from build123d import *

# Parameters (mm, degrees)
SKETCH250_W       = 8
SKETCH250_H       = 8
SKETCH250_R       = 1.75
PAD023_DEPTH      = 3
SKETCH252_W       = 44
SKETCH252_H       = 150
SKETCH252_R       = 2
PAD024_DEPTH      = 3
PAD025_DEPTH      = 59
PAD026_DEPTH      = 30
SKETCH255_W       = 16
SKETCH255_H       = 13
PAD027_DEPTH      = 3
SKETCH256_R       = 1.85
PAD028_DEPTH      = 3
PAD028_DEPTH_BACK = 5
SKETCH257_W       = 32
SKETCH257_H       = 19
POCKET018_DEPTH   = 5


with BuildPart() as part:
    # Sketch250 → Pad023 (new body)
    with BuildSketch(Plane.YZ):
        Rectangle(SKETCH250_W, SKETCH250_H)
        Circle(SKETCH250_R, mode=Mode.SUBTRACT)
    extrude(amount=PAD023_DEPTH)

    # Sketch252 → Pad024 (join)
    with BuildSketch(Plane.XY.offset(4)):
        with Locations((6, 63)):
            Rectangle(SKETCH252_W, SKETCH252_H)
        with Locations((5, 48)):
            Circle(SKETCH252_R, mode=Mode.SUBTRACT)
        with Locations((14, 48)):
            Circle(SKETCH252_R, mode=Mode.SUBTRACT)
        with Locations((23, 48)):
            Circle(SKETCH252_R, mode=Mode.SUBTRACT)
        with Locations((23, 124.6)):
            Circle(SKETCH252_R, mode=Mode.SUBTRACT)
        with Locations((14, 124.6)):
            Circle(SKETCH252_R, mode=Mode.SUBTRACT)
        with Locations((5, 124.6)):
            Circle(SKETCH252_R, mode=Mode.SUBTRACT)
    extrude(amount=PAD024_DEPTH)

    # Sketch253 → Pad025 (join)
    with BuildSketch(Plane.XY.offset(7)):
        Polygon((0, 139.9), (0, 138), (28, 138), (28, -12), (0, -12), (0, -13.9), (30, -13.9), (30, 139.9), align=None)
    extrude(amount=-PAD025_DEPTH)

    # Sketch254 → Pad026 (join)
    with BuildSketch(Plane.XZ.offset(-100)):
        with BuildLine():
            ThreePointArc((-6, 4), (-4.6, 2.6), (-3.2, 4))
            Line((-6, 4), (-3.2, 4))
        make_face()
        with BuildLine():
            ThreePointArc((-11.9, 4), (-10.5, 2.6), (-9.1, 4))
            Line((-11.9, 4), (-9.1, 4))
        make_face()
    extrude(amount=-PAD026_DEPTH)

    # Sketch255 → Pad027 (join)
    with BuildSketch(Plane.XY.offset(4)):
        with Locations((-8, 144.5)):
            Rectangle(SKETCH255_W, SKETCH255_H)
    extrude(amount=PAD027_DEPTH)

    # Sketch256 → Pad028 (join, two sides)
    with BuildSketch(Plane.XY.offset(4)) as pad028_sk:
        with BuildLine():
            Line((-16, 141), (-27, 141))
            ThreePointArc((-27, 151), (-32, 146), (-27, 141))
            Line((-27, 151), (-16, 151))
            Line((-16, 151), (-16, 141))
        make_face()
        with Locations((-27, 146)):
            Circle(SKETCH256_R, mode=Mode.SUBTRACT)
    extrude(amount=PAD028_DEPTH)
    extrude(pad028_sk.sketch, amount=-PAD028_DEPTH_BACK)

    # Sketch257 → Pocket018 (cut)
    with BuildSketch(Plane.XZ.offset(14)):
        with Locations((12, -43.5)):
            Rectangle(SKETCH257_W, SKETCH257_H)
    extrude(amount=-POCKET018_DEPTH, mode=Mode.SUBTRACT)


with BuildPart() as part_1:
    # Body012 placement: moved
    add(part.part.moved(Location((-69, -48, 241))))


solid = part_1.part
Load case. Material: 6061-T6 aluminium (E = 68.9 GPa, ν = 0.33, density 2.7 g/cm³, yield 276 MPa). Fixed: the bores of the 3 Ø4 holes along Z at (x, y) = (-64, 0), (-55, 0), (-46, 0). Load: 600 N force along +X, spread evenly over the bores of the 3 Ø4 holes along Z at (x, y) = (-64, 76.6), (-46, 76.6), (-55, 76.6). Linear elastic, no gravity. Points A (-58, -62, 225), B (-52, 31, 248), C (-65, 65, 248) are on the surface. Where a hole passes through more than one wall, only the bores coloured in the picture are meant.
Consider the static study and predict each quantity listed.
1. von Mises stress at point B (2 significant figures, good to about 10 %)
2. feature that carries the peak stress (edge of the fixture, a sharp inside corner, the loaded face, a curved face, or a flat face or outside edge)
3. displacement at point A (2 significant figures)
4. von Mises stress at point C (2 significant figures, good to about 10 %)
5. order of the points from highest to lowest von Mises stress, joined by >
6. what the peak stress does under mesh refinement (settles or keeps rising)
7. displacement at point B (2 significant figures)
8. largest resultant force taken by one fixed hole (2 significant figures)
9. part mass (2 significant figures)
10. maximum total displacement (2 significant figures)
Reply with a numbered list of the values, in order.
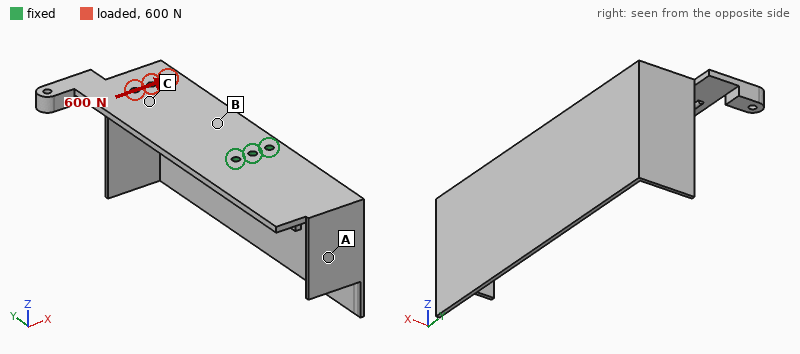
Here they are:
1. 13 MPa
2. edge of the fixture
3. 0.037 mm
4. 9.8 MPa
5. B > C > A
6. keeps rising
7. 0.033 mm
8. 2.2 kN
9. 120 g
10. 0.15 mm
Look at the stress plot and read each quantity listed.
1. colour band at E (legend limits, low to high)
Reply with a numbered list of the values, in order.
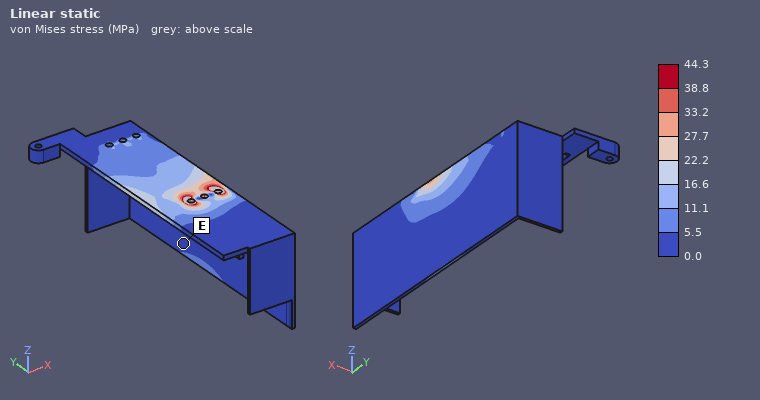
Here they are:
1. 0.0 to 5.5 MPa
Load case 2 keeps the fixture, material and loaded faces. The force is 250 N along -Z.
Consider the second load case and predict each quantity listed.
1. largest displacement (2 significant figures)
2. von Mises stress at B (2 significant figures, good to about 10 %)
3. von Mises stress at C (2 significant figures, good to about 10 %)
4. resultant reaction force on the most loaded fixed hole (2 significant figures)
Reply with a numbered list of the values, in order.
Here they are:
1. 1.6 mm
2. 26 MPa
3. 20 MPa
4. 130 N
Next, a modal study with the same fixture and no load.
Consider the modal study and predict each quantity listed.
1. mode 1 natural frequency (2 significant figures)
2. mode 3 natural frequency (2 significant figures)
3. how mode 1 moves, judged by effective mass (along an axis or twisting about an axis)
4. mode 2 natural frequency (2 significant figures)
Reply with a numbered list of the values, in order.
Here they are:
1. 310 Hz
2. 570 Hz
3. along Z
4. 380 Hz
